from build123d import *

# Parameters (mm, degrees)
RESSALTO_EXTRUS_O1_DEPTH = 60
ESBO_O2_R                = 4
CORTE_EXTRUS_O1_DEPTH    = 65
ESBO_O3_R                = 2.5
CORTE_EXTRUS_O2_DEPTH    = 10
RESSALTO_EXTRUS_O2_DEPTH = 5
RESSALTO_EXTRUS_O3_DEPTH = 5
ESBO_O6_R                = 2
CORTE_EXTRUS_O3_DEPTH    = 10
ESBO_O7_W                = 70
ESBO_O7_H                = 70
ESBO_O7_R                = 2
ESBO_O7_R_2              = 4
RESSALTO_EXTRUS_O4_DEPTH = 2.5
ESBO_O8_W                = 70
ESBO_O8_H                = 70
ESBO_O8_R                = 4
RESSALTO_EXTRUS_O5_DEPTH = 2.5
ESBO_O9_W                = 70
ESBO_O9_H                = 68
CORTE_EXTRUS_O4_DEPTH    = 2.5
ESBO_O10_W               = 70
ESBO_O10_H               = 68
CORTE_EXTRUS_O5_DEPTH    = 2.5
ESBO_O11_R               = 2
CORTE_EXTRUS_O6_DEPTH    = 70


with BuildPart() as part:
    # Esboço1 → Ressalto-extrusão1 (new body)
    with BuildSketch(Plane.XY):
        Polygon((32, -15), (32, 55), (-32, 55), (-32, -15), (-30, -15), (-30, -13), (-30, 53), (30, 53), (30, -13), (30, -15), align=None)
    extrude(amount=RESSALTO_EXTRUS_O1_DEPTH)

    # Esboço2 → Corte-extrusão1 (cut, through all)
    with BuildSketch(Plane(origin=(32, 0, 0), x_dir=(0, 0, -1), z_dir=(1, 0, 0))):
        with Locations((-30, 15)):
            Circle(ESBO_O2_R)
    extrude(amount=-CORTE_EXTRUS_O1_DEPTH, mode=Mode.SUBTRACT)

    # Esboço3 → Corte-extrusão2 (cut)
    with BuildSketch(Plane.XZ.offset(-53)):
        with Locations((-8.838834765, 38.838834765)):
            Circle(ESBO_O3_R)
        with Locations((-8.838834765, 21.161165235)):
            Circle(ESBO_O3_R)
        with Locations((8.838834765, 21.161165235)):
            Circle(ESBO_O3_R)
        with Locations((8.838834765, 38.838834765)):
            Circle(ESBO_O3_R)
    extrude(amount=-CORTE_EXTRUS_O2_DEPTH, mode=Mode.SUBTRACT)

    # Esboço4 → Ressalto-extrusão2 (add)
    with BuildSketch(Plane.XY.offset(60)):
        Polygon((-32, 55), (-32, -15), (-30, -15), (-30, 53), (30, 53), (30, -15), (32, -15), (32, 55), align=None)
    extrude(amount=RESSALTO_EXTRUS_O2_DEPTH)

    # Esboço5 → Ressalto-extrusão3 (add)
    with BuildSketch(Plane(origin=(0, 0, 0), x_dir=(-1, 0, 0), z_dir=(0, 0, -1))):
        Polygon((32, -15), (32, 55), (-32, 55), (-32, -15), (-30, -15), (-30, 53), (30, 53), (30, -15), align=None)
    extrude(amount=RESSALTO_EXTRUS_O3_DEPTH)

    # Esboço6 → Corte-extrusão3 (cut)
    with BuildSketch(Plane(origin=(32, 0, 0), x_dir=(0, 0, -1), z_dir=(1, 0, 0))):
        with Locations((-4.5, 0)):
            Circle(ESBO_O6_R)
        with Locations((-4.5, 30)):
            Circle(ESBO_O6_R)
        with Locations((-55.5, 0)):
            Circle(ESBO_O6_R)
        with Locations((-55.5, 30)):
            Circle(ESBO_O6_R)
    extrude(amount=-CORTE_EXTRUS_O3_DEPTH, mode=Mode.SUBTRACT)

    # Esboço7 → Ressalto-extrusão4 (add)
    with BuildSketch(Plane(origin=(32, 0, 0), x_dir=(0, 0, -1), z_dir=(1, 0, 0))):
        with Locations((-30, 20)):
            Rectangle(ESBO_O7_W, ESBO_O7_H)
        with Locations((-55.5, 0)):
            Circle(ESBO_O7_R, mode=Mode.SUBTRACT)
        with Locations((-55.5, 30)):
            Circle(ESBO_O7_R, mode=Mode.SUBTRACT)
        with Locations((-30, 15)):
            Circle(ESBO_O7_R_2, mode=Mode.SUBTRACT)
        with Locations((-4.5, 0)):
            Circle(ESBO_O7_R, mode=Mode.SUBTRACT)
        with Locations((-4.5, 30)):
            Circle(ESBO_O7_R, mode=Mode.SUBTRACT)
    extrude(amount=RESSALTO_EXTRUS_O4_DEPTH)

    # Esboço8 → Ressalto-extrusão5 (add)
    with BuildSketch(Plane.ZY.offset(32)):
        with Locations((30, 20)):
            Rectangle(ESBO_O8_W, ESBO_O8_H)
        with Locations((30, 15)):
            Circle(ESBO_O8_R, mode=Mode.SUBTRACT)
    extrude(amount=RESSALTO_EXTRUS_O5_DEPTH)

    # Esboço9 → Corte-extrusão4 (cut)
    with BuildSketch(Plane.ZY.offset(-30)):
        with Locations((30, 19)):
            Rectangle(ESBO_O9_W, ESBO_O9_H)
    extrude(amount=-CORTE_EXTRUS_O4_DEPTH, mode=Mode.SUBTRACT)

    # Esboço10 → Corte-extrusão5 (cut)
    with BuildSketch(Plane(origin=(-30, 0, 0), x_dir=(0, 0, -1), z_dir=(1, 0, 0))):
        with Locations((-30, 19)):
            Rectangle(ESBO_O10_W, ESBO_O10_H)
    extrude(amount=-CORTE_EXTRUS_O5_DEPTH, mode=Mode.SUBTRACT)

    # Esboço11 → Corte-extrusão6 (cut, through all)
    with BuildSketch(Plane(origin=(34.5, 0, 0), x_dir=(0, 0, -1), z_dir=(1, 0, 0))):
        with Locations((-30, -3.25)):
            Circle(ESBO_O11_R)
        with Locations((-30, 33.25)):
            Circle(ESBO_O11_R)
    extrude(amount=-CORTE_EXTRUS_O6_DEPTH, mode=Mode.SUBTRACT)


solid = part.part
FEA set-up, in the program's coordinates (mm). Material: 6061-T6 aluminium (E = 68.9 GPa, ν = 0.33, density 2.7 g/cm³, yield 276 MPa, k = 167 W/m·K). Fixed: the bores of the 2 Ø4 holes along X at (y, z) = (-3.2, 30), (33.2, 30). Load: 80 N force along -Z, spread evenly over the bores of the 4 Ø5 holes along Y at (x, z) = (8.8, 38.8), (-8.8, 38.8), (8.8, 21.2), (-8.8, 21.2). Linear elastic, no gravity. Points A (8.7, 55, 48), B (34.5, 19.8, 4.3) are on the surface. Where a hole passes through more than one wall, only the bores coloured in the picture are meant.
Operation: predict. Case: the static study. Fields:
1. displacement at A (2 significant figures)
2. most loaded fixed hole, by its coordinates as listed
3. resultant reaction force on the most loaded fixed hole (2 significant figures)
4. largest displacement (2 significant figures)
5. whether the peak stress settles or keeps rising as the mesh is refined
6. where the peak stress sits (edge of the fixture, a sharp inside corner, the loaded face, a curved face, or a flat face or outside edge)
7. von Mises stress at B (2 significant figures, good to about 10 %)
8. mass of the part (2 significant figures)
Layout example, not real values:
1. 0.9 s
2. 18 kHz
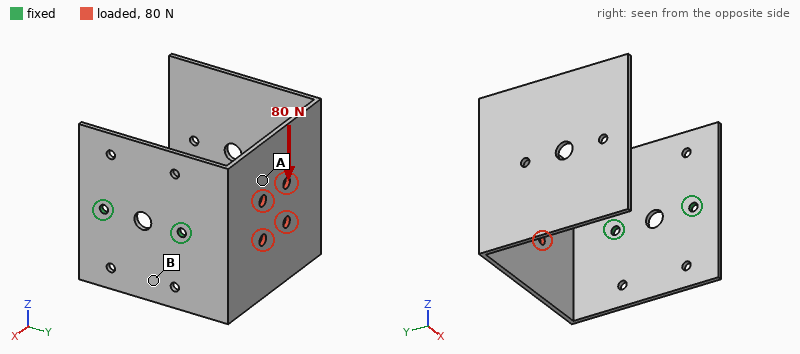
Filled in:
1. 0.37 mm
2. (33.2, 30)
3. 120 N
4. 1.2 mm
5. keeps rising
6. edge of the fixture
7. 20 MPa
8. 76 g
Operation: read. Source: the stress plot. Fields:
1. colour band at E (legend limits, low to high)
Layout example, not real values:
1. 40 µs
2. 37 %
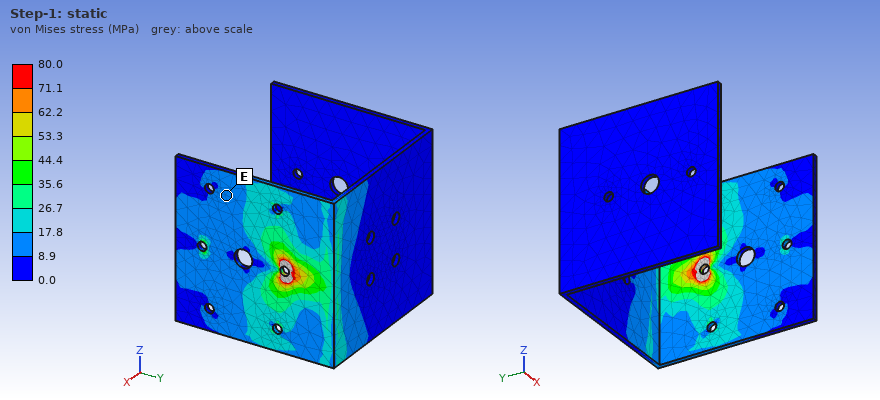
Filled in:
1. 8.9 to 17.8 MPa
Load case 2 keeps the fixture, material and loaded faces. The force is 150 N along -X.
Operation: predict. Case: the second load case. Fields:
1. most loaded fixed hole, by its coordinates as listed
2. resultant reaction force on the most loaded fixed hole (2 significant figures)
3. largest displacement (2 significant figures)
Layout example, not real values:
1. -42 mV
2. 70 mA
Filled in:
1. (33.2, 30)
2. 180 N
3. 1.1 mm
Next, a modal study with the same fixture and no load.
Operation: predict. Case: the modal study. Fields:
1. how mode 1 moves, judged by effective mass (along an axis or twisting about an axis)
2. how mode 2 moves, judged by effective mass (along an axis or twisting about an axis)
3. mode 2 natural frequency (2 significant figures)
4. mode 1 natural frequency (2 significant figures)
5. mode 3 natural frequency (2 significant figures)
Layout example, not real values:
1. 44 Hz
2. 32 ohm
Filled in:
1. along Y
2. along Z
3. 140 Hz
4. 95 Hz
5. 260 Hz
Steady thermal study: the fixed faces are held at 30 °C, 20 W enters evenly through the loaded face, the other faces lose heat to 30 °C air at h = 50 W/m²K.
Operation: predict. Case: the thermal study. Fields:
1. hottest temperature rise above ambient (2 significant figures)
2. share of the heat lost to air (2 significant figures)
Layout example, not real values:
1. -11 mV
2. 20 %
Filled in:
1. 24 K
2. 71 %
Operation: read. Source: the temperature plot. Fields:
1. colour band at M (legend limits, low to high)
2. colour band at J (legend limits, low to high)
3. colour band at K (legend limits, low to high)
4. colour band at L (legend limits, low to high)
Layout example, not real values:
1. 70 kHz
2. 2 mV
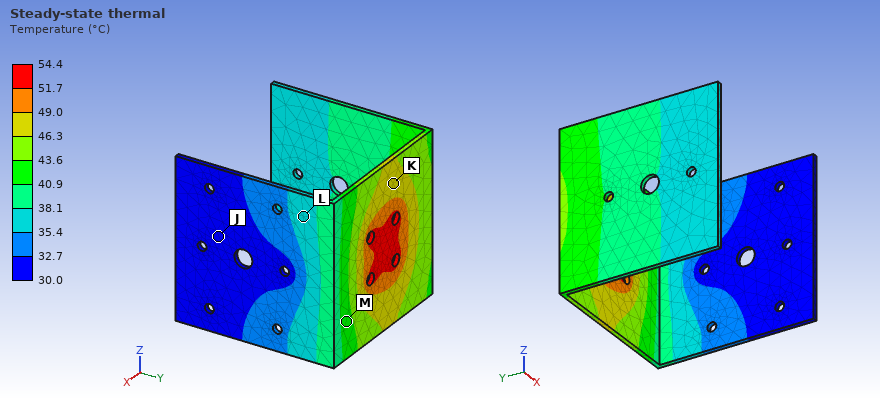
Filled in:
1. 40.9 to 43.6 °C
2. 30.0 to 32.7 °C
3. 46.3 to 49.0 °C
4. 35.4 to 38.1 °C
